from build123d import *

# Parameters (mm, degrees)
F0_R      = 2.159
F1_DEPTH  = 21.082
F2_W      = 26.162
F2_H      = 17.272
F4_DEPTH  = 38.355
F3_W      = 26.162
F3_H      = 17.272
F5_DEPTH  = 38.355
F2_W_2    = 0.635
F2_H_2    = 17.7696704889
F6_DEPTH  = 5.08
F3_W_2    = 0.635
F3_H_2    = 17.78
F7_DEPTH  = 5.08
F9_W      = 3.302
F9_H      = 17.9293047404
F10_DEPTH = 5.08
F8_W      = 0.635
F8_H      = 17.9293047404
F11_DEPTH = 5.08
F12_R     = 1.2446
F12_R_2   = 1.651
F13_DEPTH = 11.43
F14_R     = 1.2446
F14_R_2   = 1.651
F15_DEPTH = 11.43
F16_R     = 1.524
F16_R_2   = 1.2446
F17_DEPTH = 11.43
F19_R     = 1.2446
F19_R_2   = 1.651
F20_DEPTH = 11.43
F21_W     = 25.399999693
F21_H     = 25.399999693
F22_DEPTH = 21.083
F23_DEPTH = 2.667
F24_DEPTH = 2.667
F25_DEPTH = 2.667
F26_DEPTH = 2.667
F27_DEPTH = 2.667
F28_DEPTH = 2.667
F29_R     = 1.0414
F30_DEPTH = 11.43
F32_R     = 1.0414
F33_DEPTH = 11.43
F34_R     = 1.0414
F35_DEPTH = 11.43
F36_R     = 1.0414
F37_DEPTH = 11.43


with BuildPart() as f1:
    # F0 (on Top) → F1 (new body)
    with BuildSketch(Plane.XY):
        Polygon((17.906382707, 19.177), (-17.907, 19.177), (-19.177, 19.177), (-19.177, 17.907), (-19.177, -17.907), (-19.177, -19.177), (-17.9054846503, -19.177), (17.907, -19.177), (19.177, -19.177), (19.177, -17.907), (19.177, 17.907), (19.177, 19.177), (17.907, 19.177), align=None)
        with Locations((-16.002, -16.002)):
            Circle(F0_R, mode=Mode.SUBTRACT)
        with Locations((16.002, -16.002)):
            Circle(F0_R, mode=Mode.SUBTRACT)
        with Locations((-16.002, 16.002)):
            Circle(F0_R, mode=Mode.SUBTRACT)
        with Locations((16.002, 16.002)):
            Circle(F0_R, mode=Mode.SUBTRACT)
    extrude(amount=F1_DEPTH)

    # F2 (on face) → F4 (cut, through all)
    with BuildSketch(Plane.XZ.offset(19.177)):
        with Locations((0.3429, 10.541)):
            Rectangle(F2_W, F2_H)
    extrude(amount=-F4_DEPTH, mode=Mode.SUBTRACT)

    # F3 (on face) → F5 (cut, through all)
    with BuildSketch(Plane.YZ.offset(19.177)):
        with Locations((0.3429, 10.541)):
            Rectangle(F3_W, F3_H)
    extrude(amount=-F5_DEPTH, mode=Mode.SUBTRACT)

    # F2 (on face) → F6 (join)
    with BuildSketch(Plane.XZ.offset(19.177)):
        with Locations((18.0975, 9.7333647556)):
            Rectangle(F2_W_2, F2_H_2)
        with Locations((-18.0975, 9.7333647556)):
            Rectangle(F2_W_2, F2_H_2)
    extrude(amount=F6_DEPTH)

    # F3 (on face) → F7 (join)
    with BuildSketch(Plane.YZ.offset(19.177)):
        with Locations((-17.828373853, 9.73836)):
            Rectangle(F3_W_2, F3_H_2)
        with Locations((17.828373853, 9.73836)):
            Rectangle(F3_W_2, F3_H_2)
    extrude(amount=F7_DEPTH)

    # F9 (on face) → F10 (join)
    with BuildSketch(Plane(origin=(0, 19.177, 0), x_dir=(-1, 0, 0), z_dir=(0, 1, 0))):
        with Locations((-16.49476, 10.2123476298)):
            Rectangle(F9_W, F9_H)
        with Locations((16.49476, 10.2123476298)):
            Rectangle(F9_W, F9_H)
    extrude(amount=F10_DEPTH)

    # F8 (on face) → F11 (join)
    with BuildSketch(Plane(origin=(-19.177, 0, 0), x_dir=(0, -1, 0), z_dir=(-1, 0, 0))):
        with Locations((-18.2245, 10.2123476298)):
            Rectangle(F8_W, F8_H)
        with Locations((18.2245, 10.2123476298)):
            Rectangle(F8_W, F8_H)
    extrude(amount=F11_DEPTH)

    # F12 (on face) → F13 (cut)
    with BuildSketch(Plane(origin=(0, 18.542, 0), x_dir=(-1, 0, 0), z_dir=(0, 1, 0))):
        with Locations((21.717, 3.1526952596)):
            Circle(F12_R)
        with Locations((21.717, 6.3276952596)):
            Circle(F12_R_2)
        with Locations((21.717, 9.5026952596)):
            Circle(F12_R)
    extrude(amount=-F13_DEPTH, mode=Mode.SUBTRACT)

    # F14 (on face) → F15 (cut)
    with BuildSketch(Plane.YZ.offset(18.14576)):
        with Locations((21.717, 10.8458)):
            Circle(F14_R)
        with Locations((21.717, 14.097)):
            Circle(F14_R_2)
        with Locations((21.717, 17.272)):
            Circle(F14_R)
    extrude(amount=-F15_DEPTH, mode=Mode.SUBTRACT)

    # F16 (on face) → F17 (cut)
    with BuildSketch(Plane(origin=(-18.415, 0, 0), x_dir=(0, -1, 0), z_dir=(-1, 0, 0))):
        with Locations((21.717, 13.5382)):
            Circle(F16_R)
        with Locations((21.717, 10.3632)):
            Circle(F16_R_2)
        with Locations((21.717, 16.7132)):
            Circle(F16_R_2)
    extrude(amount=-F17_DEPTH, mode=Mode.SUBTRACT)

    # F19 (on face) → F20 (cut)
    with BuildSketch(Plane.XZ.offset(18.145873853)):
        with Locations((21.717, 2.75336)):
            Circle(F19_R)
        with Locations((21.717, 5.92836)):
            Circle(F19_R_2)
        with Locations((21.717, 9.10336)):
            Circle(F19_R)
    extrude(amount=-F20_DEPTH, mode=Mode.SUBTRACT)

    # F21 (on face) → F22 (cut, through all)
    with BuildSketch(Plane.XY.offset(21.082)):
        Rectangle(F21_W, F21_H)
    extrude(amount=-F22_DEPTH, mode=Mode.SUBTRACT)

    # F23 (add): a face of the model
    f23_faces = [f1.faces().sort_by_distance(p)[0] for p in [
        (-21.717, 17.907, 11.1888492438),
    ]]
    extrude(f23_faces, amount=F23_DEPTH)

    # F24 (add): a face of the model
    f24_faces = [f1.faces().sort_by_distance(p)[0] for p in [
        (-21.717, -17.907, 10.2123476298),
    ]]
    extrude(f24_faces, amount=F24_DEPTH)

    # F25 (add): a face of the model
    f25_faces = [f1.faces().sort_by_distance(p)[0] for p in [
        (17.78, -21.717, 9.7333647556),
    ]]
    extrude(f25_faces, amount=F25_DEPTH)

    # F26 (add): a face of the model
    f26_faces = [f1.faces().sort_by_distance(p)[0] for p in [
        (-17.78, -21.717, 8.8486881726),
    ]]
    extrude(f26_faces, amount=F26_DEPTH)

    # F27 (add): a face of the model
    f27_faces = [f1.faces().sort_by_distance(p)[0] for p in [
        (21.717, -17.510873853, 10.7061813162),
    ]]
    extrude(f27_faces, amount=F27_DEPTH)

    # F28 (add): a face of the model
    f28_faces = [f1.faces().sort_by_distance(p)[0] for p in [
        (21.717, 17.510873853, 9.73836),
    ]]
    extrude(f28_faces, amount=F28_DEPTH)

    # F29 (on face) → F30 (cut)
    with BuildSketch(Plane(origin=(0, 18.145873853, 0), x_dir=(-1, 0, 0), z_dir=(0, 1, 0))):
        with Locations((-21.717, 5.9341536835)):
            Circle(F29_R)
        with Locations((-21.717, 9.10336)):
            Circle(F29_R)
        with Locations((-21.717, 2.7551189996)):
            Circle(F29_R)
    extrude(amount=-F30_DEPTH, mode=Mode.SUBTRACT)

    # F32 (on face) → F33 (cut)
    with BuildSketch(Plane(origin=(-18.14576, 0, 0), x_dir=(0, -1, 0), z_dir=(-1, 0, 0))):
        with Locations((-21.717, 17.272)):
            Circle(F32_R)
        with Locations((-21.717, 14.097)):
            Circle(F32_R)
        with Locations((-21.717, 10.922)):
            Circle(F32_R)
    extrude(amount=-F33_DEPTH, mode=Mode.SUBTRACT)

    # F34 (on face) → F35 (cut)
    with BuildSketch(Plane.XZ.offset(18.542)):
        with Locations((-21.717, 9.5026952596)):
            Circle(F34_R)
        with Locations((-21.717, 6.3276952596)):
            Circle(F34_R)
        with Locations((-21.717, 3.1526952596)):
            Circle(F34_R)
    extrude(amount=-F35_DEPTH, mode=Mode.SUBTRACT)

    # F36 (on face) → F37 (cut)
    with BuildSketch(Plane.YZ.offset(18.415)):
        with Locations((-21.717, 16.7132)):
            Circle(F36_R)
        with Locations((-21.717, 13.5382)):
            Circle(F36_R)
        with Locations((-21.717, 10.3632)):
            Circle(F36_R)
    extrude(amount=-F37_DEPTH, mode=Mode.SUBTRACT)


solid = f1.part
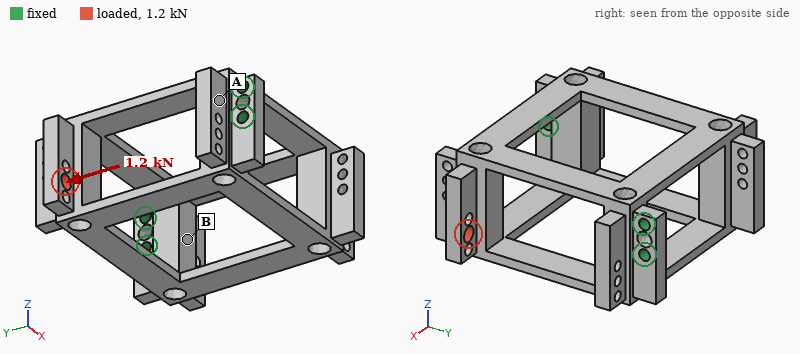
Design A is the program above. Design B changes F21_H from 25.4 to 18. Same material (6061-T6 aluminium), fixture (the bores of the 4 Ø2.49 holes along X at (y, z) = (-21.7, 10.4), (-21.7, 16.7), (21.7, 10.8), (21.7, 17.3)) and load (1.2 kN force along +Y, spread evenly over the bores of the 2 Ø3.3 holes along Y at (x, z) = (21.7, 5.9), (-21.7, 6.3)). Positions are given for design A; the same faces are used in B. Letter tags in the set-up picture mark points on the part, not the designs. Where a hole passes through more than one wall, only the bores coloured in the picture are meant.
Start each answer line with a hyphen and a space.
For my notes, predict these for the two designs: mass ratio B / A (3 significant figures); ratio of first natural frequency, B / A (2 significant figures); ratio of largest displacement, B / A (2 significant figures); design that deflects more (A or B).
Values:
- 1.11
- 1.1
- 0.91
- A
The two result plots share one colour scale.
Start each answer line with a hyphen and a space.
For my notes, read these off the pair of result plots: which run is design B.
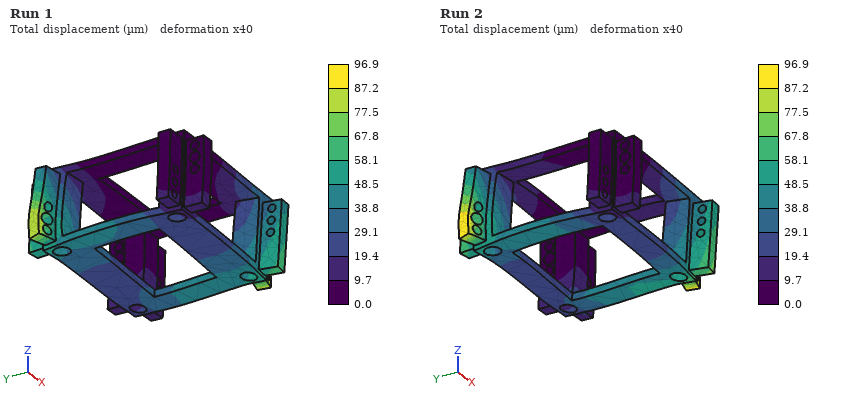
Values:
- Run 1
